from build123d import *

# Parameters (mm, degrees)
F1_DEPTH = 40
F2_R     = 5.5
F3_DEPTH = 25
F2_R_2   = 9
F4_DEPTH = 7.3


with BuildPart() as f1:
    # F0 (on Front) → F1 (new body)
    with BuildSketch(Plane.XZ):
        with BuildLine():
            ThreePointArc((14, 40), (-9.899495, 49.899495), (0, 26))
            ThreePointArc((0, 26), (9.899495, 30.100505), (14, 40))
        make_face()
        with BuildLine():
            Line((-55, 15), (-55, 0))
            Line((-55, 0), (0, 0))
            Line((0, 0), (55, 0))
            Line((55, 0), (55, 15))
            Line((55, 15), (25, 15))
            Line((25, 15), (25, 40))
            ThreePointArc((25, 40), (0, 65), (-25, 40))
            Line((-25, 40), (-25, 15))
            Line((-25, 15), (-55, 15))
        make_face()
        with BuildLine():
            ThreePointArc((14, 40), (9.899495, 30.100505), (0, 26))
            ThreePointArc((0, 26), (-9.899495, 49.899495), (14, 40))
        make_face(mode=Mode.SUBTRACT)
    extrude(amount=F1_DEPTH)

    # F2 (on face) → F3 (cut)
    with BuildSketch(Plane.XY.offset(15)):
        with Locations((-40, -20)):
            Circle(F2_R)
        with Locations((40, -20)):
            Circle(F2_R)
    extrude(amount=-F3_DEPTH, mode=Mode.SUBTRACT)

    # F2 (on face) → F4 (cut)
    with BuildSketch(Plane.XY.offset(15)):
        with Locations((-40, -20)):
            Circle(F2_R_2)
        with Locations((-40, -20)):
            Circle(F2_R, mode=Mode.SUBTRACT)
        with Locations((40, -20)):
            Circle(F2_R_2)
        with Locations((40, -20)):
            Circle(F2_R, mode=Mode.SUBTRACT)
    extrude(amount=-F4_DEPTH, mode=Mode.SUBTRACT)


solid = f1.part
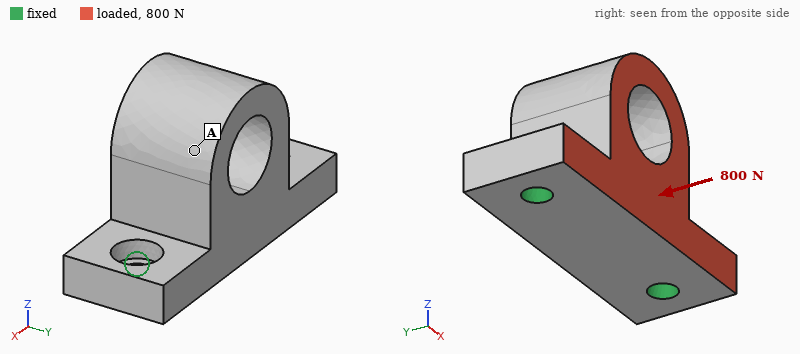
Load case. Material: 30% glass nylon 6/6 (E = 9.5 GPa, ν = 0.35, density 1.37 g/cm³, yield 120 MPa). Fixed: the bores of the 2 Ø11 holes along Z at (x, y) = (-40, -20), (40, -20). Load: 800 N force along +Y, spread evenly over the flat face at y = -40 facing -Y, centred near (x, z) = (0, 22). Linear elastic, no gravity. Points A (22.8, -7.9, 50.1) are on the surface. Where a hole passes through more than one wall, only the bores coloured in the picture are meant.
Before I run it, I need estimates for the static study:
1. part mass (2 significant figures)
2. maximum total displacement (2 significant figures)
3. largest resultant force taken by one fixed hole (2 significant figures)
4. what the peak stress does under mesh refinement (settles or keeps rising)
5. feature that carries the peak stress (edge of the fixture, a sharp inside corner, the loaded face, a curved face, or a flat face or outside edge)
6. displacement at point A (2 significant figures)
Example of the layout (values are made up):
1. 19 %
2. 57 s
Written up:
1. 170 g
2. 0.13 mm
3. 400 N
4. keeps rising
5. edge of the fixture
6. 0.095 mm
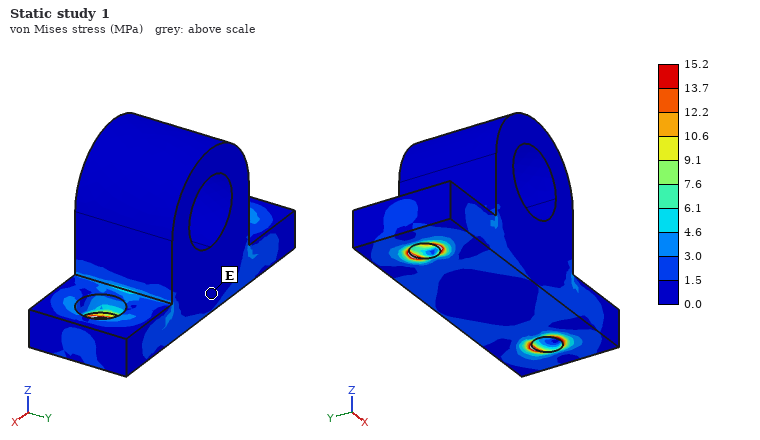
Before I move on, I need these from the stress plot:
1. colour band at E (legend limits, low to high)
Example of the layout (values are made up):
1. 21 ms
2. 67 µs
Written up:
1. 0.0 to 1.5 MPa
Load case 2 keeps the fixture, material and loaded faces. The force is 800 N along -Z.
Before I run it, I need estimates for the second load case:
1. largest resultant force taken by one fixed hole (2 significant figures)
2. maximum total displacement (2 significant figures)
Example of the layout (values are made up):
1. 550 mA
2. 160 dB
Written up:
1. 450 N
2. 0.13 mm
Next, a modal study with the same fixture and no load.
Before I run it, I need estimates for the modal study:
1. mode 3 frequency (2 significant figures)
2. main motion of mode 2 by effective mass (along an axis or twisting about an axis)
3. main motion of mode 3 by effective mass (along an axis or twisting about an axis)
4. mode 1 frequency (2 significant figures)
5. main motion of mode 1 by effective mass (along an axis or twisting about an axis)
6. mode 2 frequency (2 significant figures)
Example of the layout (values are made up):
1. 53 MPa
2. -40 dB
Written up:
1. 3600 Hz
2. along X
3. along Z
4. 1200 Hz
5. along Y
6. 3100 Hz
